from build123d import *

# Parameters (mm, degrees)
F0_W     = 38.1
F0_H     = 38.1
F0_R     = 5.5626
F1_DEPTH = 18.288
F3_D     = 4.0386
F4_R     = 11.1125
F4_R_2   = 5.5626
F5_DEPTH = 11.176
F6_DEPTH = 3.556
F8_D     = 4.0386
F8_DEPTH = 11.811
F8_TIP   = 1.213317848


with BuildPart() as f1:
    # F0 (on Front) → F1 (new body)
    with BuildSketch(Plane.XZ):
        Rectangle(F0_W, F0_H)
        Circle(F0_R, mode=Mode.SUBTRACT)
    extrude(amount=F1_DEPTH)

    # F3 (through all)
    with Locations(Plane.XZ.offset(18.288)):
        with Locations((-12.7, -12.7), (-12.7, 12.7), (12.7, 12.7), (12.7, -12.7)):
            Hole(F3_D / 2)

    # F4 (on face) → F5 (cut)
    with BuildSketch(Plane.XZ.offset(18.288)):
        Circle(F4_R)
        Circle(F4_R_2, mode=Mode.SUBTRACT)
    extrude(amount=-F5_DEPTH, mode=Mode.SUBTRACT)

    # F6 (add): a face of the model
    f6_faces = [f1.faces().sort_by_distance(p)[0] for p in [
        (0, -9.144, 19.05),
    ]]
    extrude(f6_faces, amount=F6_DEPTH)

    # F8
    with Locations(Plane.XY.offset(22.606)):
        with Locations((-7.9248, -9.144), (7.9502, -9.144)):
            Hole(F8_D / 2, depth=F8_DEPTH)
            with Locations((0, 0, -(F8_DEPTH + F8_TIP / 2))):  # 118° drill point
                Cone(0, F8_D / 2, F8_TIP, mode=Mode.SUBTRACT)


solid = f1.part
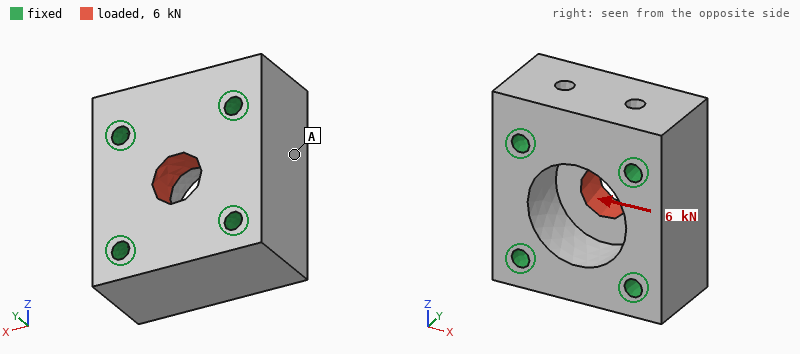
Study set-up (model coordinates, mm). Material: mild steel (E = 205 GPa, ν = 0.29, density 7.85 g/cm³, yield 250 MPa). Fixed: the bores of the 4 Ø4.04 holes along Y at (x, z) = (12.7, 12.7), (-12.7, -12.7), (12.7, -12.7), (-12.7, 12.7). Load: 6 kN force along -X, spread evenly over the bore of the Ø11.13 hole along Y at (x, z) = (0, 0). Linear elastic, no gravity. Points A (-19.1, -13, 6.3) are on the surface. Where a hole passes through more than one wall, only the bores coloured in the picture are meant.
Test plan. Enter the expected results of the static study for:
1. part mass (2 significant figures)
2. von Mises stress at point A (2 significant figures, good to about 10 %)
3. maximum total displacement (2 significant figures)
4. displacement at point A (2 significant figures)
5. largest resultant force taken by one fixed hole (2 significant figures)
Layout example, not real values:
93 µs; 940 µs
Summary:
180 g; 4.9 MPa; 1.9 µm; 0.31 µm; 1.6 kN
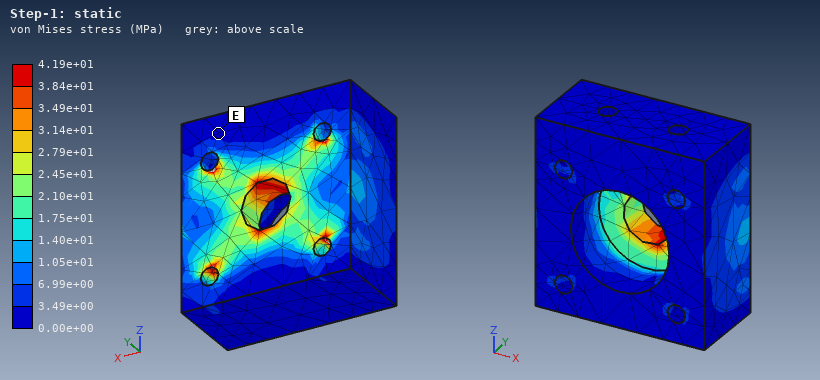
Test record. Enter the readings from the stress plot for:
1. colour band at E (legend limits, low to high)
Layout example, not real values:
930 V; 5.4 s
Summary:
0.00e+00 to 3.49e+00 MPa
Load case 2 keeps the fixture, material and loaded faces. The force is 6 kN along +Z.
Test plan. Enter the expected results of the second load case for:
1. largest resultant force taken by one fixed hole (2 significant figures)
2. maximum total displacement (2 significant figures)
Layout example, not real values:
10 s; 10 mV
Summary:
1.6 kN; 1.8 µm
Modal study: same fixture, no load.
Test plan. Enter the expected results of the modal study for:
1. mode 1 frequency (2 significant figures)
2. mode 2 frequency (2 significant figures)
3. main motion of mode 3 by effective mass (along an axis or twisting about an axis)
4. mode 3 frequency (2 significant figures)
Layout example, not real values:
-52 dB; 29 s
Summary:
45 kHz; 46 kHz; along Y; 53 kHz
